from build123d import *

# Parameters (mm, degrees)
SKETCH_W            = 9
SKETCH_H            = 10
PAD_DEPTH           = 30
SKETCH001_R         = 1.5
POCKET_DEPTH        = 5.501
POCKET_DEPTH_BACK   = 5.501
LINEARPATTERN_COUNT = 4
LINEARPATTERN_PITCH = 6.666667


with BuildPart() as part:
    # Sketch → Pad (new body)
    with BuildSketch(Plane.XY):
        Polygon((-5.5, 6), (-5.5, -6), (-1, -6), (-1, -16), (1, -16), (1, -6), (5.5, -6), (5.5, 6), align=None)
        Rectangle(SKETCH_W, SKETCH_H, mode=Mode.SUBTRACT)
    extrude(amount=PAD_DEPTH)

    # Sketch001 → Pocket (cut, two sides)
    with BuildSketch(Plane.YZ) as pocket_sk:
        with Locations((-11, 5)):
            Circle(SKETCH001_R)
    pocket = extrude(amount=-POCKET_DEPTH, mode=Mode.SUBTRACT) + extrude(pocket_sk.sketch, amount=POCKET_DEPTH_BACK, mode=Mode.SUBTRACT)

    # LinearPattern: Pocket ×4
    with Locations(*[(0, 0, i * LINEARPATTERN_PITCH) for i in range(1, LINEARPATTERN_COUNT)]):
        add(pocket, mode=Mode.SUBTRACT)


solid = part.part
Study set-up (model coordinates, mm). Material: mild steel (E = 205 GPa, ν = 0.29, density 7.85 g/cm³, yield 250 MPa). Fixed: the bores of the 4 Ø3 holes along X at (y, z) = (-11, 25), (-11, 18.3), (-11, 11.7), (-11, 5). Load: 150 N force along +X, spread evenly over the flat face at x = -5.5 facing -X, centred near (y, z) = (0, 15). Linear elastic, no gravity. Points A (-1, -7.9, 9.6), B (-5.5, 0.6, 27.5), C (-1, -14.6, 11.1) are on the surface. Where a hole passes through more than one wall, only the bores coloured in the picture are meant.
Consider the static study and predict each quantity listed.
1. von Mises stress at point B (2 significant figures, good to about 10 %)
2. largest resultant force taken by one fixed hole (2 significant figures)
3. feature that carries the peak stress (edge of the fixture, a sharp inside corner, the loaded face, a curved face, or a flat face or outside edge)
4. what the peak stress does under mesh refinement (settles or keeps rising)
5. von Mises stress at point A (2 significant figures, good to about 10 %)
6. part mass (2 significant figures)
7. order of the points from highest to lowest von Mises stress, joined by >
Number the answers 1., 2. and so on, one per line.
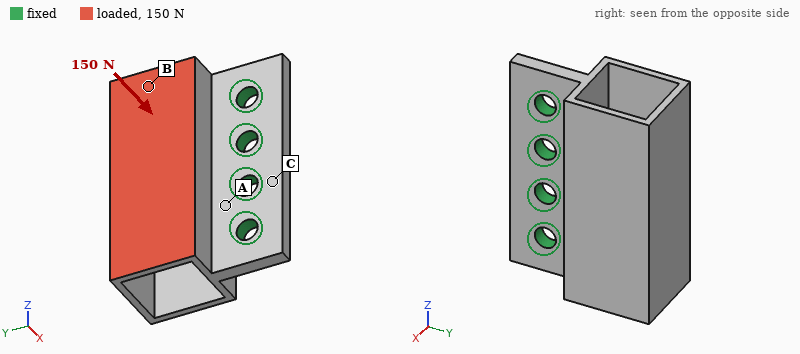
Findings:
1. 26 MPa
2. 38 N
3. edge of the fixture
4. keeps rising
5. 52 MPa
6. 14 g
7. A > B > C
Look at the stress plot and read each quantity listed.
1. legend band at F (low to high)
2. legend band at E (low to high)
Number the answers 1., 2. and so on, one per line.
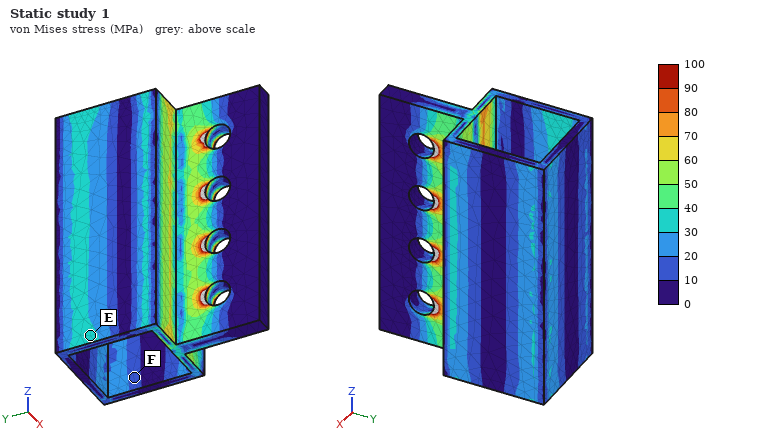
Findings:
1. 10 to 20 MPa
2. 30 to 40 MPa
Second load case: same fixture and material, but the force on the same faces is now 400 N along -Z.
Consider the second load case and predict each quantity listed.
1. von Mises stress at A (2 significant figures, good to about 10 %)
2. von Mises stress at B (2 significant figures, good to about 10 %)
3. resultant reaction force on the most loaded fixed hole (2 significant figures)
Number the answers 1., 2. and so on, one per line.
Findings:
1. 23 MPa
2. 14 MPa
3. 220 N
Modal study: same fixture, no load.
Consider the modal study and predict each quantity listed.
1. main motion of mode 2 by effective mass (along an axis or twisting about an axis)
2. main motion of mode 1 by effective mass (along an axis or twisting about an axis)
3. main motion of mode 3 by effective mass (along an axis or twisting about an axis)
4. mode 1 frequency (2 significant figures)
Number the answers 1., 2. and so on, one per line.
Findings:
1. along Z
2. along X
3. twisting about Y
4. 3000 Hz
